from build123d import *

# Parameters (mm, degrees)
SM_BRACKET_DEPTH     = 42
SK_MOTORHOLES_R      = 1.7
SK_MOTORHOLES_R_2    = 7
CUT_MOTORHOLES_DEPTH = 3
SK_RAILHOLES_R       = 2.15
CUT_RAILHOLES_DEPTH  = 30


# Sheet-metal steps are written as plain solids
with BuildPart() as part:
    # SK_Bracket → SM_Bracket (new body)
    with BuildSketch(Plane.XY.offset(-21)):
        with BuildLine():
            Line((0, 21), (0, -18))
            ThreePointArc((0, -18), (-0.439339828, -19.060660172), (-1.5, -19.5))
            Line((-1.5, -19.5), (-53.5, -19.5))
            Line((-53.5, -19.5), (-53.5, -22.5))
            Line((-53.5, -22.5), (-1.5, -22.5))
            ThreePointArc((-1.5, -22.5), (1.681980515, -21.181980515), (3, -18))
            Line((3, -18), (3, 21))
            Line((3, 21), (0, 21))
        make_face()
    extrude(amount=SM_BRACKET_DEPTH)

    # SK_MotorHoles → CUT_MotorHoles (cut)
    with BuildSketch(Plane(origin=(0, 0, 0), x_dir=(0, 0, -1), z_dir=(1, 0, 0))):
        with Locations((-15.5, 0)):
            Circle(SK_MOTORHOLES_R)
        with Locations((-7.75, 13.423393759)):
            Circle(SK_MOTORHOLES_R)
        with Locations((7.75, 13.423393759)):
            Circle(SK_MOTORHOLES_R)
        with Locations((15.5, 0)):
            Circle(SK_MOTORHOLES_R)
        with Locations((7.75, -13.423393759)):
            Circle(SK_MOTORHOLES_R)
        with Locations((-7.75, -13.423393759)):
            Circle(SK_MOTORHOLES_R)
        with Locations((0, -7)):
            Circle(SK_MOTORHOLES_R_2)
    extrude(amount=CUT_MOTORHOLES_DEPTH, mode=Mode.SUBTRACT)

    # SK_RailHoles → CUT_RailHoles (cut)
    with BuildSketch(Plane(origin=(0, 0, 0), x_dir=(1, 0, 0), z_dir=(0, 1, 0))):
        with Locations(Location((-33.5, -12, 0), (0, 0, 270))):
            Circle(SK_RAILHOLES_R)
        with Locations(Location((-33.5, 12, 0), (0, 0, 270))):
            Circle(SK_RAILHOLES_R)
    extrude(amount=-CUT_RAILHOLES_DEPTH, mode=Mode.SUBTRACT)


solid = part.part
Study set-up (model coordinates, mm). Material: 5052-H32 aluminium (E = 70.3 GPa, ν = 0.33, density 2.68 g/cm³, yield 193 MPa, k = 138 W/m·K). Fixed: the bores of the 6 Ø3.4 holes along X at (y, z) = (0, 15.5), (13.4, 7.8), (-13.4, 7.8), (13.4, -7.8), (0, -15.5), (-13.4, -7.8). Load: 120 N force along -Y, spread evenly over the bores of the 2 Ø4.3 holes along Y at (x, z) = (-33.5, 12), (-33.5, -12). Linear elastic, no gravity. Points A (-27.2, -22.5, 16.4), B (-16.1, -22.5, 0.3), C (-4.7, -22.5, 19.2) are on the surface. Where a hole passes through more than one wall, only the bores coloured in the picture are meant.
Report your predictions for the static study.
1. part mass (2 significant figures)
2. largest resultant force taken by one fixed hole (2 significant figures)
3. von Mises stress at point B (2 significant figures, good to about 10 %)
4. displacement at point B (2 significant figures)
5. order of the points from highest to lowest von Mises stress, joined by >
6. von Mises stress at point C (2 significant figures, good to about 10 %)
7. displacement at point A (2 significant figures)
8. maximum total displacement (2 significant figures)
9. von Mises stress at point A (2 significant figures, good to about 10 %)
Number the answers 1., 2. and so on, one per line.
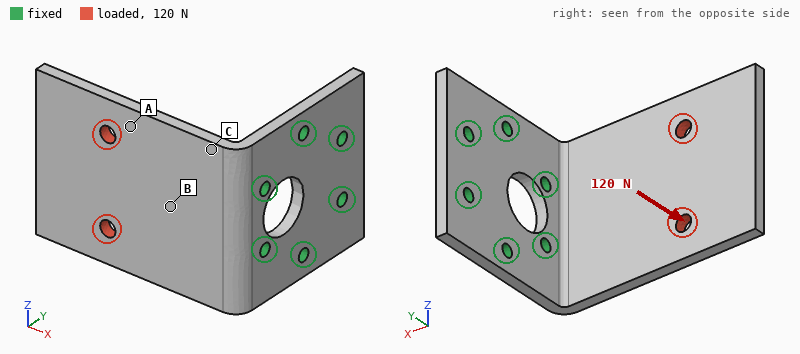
1. 30 g
2. 82 N
3. 29 MPa
4. 0.16 mm
5. C > B > A
6. 54 MPa
7. 0.30 mm
8. 0.68 mm
9. 13 MPa
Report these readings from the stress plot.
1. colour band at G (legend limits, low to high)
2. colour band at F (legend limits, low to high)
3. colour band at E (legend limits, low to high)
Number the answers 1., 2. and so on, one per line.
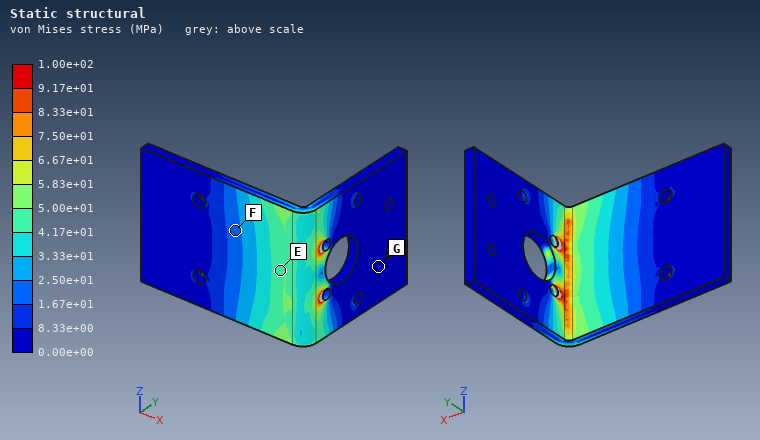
1. 0.00e+00 to 8.33e+00 MPa
2. 1.67e+01 to 2.50e+01 MPa
3. 4.17e+01 to 5.00e+01 MPa
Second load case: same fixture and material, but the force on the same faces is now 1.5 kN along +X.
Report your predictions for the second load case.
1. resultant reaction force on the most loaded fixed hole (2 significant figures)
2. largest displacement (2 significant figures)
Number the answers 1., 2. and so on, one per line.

1. 830 N
2. 0.41 mm
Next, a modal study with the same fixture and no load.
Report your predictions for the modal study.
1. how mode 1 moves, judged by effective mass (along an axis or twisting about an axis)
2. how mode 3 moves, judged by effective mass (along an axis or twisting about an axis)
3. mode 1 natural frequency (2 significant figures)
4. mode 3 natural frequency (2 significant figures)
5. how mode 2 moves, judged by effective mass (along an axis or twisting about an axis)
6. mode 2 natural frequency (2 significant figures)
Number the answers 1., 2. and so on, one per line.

1. along Y
2. along Z
3. 690 Hz
4. 2800 Hz
5. along Z
6. 2100 Hz
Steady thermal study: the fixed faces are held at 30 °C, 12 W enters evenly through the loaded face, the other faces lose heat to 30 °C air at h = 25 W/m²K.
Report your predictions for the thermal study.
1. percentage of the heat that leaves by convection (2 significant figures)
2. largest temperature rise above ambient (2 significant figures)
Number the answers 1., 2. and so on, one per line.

1. 20 %
2. 27 K
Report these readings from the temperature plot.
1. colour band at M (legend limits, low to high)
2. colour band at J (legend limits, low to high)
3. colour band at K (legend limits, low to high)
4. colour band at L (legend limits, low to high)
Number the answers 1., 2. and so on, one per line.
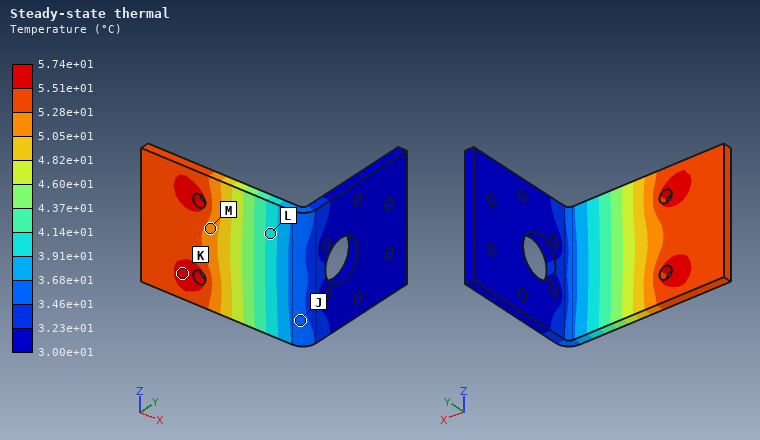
1. 5.05e+01 to 5.28e+01 °C
2. 3.46e+01 to 3.68e+01 °C
3. 5.51e+01 to 5.74e+01 °C
4. 3.91e+01 to 4.14e+01 °C
